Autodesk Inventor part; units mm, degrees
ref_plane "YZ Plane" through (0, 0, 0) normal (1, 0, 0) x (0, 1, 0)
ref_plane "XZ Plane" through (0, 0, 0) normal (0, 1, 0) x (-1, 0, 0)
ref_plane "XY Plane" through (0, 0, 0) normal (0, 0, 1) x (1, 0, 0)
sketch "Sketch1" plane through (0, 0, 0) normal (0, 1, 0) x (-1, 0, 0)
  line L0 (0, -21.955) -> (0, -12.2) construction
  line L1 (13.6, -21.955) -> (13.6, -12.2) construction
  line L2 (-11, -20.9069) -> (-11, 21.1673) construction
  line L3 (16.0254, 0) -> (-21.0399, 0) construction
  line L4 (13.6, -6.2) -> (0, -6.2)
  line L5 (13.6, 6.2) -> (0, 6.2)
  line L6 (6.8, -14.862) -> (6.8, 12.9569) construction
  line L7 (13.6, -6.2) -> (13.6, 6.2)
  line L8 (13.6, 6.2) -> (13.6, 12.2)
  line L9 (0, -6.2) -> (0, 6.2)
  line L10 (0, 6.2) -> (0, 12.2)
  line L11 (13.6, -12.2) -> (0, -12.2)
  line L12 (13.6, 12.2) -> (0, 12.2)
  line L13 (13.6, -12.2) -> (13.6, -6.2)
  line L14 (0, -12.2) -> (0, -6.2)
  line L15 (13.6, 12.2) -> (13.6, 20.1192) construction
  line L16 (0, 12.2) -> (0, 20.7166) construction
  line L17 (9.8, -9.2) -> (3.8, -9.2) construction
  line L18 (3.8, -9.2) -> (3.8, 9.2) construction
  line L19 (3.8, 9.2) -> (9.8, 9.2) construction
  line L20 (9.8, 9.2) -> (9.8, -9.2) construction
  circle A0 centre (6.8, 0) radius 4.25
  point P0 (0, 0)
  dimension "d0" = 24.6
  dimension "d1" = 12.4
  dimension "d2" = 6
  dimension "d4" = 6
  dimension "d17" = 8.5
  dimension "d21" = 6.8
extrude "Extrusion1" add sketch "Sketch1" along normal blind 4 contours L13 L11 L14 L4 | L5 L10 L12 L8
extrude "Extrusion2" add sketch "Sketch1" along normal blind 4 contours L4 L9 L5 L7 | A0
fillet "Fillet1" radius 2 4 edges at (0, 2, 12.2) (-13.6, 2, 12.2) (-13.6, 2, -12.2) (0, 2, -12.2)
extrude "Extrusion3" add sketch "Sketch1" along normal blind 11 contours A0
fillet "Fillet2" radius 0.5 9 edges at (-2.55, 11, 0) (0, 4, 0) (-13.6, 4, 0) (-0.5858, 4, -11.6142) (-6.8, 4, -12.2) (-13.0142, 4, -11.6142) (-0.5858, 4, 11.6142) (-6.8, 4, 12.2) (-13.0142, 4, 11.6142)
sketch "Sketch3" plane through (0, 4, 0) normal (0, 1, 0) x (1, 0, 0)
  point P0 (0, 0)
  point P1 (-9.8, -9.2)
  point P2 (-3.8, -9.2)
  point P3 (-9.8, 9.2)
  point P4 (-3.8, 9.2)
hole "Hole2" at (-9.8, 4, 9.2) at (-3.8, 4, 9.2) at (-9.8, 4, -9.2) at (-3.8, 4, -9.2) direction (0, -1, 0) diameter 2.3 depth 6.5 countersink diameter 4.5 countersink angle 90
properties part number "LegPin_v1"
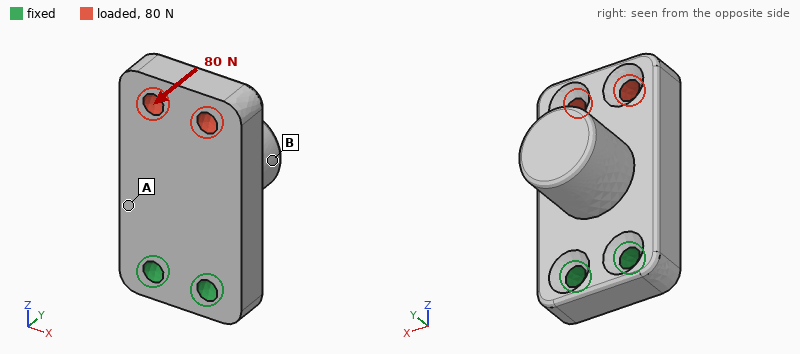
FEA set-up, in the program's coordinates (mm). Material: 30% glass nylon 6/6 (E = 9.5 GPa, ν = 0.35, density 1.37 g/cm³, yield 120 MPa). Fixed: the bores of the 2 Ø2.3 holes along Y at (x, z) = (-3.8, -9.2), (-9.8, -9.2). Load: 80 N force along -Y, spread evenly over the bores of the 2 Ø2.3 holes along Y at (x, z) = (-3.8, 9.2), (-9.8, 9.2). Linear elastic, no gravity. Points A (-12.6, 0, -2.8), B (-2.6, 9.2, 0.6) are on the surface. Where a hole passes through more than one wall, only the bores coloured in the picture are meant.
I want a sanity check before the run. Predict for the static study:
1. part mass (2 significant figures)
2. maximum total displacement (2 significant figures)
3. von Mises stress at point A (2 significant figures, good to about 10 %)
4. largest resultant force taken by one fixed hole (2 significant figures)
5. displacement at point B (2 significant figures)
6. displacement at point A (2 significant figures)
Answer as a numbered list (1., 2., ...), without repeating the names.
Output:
1. 2.2 g
2. 0.31 mm
3. 21 MPa
4. 40 N
5. 0.15 mm
6. 0.055 mm
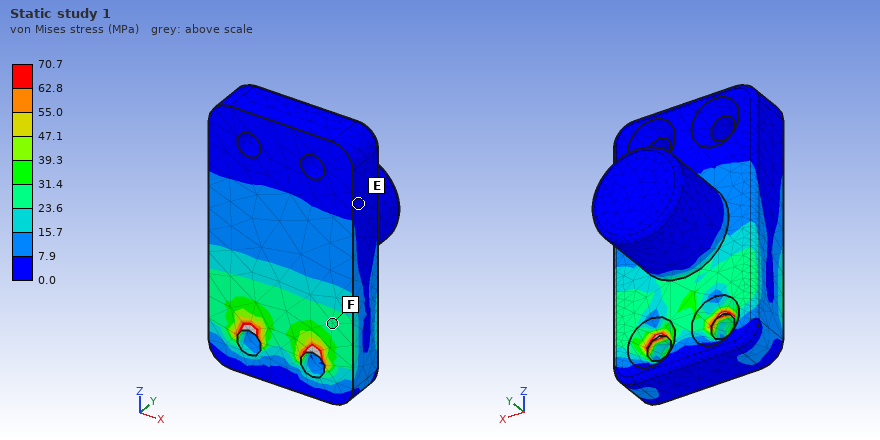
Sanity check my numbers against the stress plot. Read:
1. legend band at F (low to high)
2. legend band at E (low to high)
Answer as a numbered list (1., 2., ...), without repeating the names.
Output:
1. 23.6 to 31.4 MPa
2. 0.0 to 7.9 MPa
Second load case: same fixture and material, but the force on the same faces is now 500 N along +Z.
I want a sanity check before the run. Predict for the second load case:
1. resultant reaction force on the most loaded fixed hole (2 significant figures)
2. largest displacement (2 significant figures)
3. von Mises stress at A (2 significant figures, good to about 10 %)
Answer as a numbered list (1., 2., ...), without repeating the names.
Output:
1. 250 N
2. 84 µm
3. 15 MPa
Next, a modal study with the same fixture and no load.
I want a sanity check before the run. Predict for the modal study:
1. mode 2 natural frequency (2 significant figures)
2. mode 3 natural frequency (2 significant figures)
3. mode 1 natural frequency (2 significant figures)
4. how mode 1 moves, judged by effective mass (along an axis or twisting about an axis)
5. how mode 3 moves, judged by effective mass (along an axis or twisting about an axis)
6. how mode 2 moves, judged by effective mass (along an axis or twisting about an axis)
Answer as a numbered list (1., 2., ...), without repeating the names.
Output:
1. 8300 Hz
2. 9700 Hz
3. 3300 Hz
4. along Y
5. twisting about Z
6. along X
